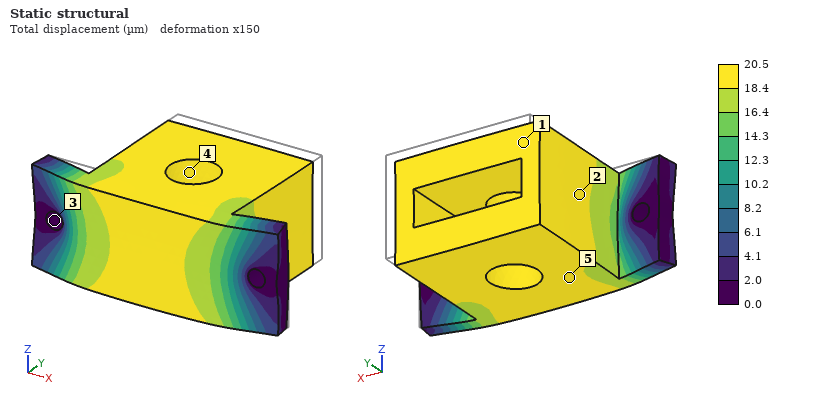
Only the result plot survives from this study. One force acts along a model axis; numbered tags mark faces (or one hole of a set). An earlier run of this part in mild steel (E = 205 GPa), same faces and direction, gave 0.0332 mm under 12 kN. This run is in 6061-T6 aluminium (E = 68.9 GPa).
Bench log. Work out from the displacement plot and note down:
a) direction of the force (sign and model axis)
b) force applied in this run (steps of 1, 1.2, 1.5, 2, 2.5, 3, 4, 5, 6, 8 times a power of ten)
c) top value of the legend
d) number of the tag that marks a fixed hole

-Y
2.5 kN
20.5 µm
3
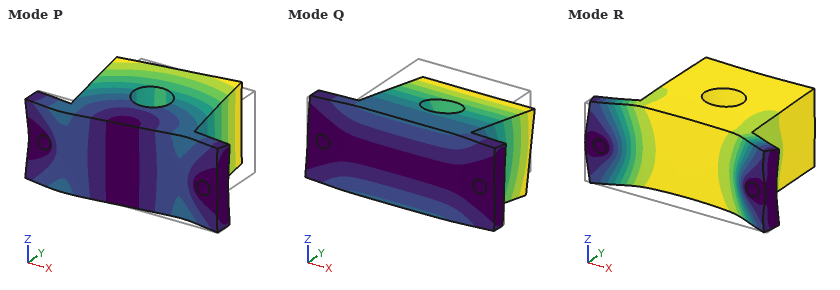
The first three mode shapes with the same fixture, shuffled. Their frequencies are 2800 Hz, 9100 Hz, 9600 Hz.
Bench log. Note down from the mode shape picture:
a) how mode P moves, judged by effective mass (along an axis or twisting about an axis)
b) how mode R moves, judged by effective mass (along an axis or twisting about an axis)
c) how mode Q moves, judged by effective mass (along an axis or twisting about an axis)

along X
along Y
along Z
